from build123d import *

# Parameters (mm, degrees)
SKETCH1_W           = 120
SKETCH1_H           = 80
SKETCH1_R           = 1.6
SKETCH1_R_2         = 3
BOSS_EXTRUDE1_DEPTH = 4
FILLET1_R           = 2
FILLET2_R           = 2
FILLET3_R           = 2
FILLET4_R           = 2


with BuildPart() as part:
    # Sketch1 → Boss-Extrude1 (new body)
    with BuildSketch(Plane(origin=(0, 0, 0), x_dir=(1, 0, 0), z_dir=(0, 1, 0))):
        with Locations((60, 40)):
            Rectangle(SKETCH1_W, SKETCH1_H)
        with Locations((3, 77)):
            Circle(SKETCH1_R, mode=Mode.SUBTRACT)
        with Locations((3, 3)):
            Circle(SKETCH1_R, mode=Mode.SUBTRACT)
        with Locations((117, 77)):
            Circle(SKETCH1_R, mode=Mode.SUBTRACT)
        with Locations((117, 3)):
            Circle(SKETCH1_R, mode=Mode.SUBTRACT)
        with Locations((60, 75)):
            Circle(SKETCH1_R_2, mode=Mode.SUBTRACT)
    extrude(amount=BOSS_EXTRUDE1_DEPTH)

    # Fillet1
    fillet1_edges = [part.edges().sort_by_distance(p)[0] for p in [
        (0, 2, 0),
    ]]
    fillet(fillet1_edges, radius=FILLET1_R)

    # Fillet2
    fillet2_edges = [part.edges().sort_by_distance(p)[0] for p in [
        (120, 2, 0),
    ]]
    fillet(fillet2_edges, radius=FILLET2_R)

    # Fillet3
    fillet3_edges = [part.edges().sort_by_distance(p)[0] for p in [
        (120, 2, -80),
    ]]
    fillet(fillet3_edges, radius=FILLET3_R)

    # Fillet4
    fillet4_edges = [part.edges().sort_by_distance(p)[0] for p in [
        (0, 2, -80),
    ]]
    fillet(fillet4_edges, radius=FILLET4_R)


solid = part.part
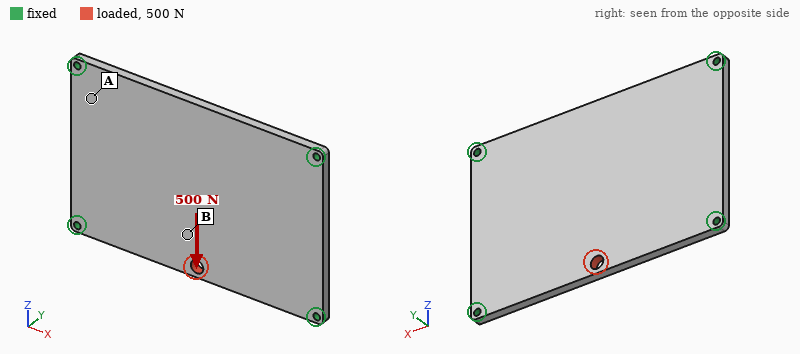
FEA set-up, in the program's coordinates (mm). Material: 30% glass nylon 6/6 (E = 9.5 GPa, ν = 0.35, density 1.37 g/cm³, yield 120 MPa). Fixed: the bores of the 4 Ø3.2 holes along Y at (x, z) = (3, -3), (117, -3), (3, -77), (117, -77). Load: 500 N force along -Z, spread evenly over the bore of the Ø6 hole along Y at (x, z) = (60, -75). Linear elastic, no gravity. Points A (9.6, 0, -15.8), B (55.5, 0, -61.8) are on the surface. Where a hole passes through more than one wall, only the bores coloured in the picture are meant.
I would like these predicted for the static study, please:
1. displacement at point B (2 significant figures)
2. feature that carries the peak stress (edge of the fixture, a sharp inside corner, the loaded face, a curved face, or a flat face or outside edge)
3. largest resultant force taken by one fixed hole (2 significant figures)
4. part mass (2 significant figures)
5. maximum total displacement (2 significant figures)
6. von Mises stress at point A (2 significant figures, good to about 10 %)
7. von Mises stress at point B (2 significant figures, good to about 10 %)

23 µm
a flat face or outside edge
160 N
52 g
42 µm
2.1 MPa
4.3 MPa
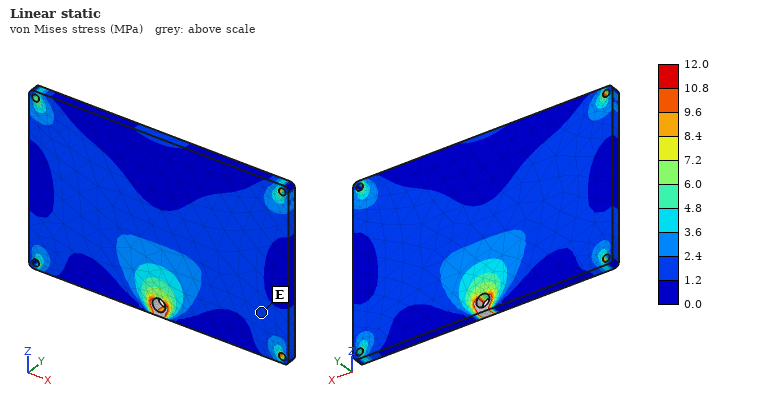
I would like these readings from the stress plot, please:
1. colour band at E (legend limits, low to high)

1.2 to 2.4 MPa
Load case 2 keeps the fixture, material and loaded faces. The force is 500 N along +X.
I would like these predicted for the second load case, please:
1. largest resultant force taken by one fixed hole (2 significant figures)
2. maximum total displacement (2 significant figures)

170 N
27 µm
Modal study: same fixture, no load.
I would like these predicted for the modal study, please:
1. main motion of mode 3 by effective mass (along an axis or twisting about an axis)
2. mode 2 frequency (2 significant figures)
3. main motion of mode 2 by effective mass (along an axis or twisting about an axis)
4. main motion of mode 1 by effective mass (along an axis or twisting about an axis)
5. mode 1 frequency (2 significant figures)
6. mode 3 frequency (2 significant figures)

twisting about Z
1100 Hz
twisting about X
along Y
600 Hz
1500 Hz
